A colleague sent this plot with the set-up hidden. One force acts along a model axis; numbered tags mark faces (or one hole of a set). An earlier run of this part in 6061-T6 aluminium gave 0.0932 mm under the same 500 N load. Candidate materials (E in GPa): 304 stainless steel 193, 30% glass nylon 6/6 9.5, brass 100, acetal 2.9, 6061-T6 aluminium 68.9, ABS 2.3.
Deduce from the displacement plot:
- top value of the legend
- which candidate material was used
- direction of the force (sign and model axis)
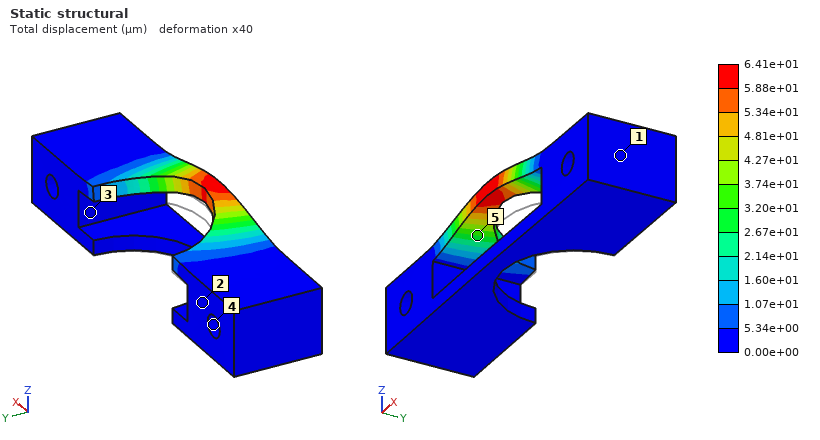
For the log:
6.41e+01 µm
brass
+Z
